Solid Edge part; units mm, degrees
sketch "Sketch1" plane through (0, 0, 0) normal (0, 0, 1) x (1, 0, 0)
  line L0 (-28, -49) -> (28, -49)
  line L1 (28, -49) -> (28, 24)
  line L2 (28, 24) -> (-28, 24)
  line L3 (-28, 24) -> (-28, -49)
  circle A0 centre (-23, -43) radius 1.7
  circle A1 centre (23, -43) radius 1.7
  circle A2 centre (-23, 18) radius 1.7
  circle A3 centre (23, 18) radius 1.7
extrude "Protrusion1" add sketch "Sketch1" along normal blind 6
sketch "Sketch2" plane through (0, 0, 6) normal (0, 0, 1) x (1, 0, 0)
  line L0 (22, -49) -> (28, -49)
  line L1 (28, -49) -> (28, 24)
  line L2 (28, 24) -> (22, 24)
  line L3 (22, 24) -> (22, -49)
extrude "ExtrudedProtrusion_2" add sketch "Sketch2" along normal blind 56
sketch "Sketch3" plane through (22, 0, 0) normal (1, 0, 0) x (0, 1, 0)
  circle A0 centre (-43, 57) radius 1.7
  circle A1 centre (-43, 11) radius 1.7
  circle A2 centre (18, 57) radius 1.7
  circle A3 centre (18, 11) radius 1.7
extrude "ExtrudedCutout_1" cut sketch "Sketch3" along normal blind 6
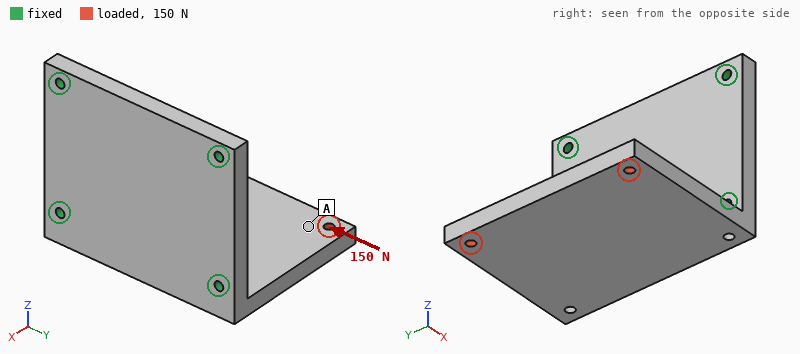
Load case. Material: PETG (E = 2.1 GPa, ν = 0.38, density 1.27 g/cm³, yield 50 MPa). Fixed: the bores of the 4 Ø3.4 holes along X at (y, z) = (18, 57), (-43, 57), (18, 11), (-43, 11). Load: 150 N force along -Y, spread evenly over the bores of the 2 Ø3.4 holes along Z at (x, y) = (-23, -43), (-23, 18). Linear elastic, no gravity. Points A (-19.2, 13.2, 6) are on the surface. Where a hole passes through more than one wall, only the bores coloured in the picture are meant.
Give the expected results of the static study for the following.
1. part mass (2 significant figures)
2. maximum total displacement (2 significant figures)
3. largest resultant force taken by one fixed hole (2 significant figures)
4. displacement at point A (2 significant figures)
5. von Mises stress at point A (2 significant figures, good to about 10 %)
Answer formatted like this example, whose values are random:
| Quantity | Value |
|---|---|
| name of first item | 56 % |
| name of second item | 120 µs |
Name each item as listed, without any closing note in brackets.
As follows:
| Quantity | Value |
|---|---|
| part mass | 62 g |
| maximum total displacement | 0.18 mm |
| largest resultant force taken by one fixed hole | 140 N |
| displacement at point A | 0.13 mm |
| von Mises stress at point A | 1.1 MPa |
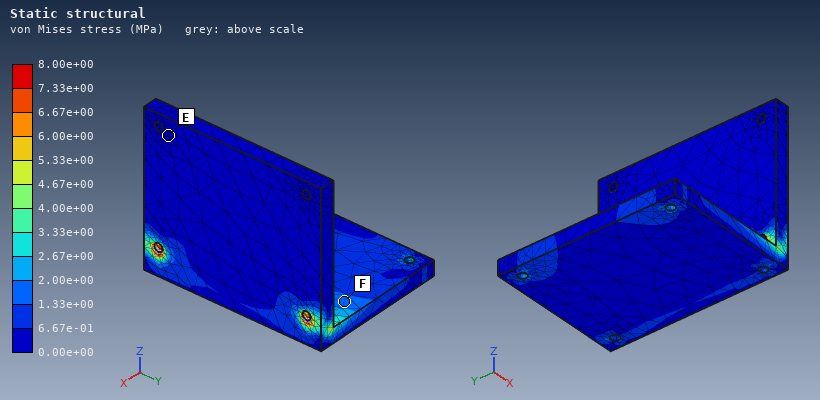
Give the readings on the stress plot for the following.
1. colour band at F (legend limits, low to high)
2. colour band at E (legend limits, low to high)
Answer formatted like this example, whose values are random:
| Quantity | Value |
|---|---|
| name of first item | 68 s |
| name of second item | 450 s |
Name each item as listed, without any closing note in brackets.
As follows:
| Quantity | Value |
|---|---|
| colour band at F | 1.33e+00 to 2.00e+00 MPa |
| colour band at E | 0.00e+00 to 6.67e-01 MPa |
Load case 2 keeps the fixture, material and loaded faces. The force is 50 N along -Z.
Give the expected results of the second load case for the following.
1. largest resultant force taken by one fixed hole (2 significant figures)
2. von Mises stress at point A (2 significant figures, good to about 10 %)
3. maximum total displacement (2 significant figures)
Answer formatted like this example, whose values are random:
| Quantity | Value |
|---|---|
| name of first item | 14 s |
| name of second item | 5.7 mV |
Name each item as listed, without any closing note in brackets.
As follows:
| Quantity | Value |
|---|---|
| largest resultant force taken by one fixed hole | 19 N |
| von Mises stress at point A | 1.3 MPa |
| maximum total displacement | 1.2 mm |
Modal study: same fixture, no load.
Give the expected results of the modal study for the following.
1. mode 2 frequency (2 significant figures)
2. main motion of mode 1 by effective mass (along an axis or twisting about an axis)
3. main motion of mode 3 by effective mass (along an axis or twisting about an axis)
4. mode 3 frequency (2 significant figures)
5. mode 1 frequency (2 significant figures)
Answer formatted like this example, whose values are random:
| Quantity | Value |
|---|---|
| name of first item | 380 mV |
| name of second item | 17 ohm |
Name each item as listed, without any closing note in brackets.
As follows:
| Quantity | Value |
|---|---|
| mode 2 frequency | 750 Hz |
| main motion of mode 1 by effective mass | along Z |
| main motion of mode 3 by effective mass | along Y |
| mode 3 frequency | 1600 Hz |
| mode 1 frequency | 340 Hz |
